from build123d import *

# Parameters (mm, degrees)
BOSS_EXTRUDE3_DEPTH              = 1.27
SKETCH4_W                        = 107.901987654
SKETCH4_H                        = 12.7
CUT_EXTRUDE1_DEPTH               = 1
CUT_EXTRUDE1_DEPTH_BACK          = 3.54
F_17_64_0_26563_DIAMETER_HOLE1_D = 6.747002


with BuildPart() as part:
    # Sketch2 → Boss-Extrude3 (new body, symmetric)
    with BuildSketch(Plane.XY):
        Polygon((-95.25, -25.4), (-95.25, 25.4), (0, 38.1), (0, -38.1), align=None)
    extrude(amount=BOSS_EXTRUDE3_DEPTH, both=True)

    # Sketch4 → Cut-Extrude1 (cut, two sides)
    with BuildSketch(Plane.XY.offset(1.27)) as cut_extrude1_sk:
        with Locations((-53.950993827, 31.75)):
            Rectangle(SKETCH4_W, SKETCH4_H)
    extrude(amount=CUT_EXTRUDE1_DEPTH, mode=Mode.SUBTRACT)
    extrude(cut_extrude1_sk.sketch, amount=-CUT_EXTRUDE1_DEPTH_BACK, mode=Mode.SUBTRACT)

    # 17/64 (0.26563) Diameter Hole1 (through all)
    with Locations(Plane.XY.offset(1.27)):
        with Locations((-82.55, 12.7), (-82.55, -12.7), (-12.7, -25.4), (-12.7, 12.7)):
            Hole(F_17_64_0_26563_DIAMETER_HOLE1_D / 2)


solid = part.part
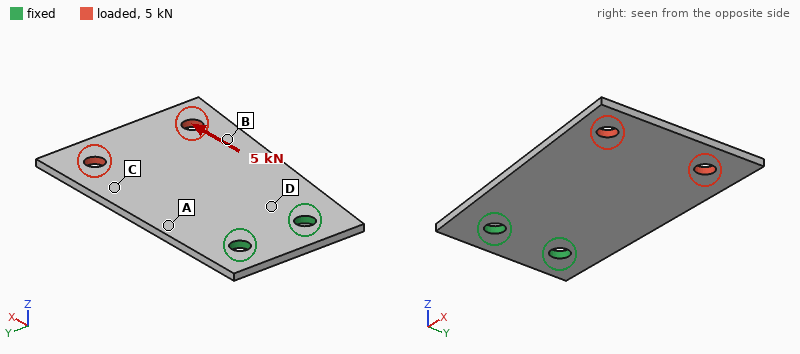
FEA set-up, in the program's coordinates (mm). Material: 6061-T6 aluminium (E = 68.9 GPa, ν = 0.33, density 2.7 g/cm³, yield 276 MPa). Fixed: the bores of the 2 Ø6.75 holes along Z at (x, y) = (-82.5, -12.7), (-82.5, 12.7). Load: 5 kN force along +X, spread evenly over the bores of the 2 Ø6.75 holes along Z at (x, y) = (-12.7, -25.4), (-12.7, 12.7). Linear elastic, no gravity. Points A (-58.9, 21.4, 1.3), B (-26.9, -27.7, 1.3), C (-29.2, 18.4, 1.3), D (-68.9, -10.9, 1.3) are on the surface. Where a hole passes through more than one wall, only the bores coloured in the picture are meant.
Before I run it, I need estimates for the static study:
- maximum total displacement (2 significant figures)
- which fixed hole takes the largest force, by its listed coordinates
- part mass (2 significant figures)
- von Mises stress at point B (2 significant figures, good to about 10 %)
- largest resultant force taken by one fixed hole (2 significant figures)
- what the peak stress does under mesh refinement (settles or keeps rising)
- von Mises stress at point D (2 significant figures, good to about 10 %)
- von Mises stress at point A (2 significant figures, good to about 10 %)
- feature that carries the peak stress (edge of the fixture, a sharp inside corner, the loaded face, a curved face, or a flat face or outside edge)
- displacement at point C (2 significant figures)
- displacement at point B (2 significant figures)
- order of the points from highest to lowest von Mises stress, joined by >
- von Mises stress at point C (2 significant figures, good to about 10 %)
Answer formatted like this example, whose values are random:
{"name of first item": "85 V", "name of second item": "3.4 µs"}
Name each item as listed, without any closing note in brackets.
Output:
{"maximum total displacement": "77 µm", "which fixed hole takes the largest force, by its listed coordinates": "(-82.5, -12.7)", "part mass": "36 g", "von Mises stress at point B": "44 MPa", "largest resultant force taken by one fixed hole": "3.6 kN", "what the peak stress does under mesh refinement": "keeps rising", "von Mises stress at point D": "56 MPa", "von Mises stress at point A": "20 MPa", "feature that carries the peak stress": "edge of the fixture", "displacement at point C": "29 µm", "displacement at point B": "57 µm", "order of the points from highest to lowest von Mises stress, joined by >": "D > B > C > A", "von Mises stress at point C": "32 MPa"}
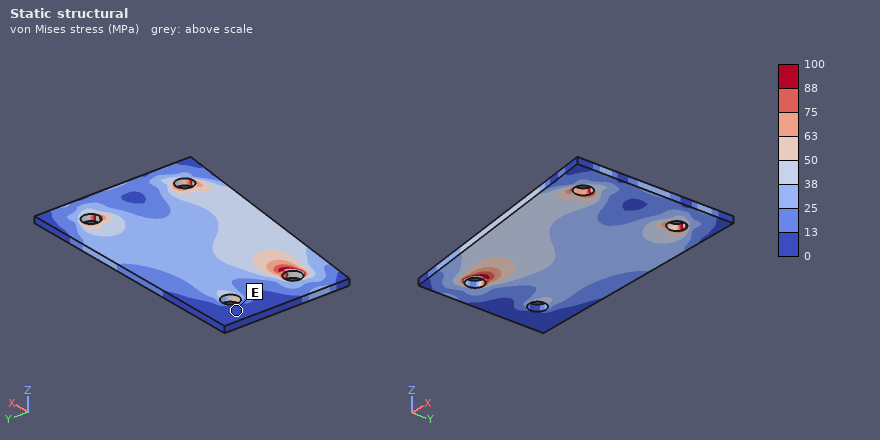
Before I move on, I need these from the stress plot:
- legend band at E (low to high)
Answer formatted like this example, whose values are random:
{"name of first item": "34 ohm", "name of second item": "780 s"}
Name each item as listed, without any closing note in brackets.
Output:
{"legend band at E": "0 to 13 MPa"}
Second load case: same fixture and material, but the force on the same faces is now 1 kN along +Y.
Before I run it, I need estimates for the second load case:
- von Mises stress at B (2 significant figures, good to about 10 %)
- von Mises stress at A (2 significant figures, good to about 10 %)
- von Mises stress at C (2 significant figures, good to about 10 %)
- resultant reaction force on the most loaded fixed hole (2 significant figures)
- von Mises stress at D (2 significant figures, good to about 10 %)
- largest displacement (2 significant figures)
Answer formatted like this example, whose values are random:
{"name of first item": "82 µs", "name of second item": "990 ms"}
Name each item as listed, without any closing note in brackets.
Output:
{"von Mises stress at B": "8.9 MPa", "von Mises stress at A": "31 MPa", "von Mises stress at C": "12 MPa", "resultant reaction force on the most loaded fixed hole": "2.4 kN", "von Mises stress at D": "34 MPa", "largest displacement": "0.12 mm"}
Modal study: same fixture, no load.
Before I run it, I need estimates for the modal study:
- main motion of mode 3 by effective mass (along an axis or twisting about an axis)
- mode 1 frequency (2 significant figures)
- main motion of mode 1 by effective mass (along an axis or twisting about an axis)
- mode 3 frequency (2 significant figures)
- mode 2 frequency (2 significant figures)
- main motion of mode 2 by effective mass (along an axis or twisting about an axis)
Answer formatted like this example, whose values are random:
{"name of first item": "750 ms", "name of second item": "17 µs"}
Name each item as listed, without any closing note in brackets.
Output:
{"main motion of mode 3 by effective mass": "along Z", "mode 1 frequency": "310 Hz", "main motion of mode 1 by effective mass": "along Z", "mode 3 frequency": "1900 Hz", "mode 2 frequency": "910 Hz", "main motion of mode 2 by effective mass": "twisting about X"}
